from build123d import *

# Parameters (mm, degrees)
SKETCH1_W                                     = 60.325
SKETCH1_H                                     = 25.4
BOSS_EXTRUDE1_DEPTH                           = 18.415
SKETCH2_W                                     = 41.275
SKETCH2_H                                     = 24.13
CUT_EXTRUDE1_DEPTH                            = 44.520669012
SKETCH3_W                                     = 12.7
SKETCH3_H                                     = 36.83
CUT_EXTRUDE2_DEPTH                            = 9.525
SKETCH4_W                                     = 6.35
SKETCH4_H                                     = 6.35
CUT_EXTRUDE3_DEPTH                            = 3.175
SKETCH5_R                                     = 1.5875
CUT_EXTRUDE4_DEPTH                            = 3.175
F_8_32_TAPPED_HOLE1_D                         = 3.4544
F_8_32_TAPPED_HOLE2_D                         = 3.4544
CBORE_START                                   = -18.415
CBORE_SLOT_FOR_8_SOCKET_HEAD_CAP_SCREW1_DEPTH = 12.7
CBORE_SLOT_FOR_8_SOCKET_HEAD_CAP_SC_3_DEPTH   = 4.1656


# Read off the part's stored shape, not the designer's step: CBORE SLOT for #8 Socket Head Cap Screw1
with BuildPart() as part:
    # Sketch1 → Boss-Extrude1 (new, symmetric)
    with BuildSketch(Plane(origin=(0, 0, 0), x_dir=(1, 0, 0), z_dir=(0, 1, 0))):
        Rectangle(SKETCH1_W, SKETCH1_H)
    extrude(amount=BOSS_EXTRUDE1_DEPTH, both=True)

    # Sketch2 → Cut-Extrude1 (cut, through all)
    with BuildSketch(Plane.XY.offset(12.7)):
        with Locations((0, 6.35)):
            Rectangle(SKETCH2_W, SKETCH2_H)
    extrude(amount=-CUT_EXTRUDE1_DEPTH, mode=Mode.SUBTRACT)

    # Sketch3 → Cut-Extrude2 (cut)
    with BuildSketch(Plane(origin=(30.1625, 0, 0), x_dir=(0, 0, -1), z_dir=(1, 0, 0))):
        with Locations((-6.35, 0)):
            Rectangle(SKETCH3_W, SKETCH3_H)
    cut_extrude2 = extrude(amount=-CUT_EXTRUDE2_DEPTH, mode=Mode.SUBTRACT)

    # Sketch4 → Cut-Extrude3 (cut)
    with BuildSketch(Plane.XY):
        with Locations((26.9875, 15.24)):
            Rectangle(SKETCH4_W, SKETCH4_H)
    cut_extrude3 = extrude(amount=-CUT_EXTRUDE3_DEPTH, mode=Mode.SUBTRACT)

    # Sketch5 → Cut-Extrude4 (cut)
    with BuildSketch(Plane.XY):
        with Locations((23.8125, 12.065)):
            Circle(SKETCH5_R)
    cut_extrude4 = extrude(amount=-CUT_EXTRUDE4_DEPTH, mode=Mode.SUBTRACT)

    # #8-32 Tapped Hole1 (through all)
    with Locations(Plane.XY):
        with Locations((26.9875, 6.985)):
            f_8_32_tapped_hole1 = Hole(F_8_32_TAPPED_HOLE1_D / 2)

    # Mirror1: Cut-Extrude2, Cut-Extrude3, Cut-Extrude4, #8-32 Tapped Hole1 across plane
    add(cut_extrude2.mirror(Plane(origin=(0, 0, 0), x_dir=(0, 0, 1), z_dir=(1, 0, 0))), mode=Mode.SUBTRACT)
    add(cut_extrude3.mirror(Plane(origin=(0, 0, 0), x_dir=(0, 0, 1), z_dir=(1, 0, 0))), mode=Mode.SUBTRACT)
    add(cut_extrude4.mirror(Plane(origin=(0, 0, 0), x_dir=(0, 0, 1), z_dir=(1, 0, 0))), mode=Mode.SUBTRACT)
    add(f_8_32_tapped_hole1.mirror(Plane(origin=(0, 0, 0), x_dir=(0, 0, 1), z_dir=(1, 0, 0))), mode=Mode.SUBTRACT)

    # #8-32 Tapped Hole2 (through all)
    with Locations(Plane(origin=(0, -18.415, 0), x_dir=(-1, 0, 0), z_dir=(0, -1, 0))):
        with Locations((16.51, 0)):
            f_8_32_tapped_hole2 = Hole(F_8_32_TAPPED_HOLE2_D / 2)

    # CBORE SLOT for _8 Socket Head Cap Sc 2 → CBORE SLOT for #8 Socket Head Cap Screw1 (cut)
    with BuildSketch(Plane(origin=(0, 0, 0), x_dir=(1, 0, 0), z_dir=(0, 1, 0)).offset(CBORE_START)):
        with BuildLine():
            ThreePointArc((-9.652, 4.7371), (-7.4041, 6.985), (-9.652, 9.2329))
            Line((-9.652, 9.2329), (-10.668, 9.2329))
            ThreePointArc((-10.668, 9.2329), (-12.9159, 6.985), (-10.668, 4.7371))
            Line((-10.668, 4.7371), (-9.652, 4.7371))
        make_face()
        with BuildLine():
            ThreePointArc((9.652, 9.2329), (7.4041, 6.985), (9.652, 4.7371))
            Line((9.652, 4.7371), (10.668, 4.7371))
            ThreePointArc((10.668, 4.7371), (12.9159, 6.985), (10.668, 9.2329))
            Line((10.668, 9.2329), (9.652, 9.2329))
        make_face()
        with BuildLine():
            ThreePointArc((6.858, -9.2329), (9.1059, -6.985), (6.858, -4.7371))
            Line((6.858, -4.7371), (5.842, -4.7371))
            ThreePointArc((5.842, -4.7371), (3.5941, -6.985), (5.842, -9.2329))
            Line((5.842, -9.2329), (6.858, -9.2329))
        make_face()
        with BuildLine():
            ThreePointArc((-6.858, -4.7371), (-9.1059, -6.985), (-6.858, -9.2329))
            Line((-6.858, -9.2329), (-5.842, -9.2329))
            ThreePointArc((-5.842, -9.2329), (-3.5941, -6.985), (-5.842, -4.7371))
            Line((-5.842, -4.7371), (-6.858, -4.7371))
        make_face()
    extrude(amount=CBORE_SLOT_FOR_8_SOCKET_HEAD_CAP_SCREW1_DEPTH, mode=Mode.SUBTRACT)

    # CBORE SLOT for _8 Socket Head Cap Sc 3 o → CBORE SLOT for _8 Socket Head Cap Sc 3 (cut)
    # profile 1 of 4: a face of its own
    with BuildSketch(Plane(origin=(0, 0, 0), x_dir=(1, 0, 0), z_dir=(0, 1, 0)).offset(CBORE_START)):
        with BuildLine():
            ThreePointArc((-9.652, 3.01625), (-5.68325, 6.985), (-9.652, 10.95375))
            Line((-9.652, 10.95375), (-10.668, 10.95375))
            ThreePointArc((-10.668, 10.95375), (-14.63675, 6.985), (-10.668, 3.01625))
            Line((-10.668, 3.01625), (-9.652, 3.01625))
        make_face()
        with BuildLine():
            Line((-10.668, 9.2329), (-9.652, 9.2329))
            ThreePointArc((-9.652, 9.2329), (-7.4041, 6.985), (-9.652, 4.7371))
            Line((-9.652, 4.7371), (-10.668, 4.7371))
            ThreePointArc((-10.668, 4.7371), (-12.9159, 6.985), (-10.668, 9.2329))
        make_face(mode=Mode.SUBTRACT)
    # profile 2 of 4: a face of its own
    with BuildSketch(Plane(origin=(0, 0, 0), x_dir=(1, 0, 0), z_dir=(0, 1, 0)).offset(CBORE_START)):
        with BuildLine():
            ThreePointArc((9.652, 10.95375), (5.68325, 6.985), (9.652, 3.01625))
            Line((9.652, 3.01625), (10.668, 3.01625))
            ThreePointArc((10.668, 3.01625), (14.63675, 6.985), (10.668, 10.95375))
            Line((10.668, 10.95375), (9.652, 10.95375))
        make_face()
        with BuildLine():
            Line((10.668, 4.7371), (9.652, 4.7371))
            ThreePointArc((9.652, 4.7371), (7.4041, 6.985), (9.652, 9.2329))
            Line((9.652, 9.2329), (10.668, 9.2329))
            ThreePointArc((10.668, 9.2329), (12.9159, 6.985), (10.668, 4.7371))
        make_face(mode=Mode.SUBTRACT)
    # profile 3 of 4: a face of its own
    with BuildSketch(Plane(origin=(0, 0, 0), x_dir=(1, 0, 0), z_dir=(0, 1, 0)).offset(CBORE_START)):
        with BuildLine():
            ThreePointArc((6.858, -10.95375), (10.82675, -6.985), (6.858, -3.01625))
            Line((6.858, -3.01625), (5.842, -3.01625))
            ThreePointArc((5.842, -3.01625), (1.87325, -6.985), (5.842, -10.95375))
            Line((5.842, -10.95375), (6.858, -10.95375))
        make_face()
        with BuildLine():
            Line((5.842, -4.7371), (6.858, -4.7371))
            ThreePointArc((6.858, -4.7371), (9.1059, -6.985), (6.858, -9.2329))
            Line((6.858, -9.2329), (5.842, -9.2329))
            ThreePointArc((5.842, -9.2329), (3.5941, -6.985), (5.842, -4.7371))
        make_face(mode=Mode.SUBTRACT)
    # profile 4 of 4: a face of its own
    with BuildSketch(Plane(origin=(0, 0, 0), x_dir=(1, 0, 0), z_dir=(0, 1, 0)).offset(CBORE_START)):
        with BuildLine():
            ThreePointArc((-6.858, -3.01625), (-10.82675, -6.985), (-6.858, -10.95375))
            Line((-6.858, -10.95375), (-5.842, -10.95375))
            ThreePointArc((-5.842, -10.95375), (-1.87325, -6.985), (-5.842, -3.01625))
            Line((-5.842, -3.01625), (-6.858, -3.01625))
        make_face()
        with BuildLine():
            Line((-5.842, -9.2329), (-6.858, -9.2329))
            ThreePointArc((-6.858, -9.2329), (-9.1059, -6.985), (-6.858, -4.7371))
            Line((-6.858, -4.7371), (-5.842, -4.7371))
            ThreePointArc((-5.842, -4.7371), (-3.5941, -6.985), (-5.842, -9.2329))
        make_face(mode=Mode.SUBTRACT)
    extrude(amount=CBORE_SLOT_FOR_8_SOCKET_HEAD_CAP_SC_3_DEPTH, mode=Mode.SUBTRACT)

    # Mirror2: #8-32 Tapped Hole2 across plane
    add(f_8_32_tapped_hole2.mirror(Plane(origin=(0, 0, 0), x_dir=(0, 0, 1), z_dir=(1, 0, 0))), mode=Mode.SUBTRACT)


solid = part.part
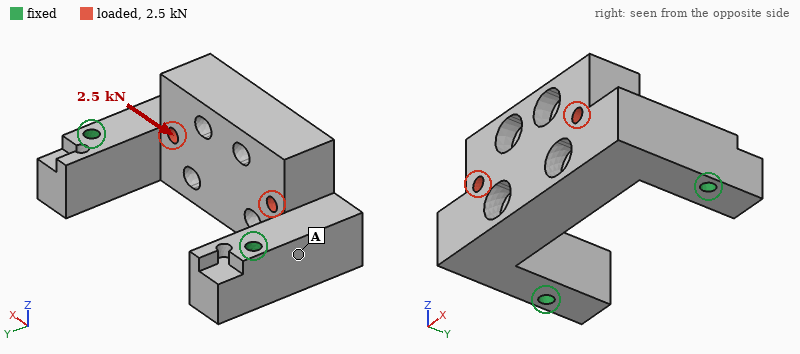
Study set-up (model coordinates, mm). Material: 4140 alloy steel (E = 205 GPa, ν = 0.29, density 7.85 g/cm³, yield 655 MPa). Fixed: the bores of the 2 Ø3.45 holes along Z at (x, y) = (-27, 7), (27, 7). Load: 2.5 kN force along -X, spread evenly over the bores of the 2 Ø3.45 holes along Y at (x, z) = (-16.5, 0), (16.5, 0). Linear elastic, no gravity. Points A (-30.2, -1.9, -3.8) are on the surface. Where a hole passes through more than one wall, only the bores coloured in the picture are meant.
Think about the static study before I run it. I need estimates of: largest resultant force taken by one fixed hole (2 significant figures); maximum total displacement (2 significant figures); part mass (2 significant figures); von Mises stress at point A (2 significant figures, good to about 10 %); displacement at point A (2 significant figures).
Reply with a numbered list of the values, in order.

1. 1.4 kN
2. 9.7 µm
3. 160 g
4. 12 MPa
5. 4.4 µm
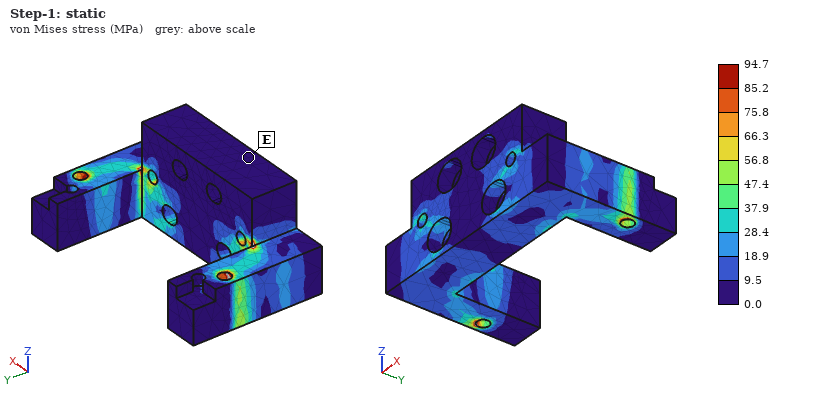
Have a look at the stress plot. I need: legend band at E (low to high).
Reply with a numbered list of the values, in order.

1. 0.0 to 9.5 MPa
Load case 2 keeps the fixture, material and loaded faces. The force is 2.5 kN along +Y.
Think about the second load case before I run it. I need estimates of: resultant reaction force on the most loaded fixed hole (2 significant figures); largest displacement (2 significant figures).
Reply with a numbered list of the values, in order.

1. 1.4 kN
2. 16 µm
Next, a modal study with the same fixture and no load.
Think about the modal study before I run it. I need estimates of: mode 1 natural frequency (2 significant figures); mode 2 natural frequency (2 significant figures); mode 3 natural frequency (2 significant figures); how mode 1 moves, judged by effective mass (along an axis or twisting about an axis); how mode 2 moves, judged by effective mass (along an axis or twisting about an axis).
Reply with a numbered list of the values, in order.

1. 5500 Hz
2. 7900 Hz
3. 11 kHz
4. along Z
5. along X
